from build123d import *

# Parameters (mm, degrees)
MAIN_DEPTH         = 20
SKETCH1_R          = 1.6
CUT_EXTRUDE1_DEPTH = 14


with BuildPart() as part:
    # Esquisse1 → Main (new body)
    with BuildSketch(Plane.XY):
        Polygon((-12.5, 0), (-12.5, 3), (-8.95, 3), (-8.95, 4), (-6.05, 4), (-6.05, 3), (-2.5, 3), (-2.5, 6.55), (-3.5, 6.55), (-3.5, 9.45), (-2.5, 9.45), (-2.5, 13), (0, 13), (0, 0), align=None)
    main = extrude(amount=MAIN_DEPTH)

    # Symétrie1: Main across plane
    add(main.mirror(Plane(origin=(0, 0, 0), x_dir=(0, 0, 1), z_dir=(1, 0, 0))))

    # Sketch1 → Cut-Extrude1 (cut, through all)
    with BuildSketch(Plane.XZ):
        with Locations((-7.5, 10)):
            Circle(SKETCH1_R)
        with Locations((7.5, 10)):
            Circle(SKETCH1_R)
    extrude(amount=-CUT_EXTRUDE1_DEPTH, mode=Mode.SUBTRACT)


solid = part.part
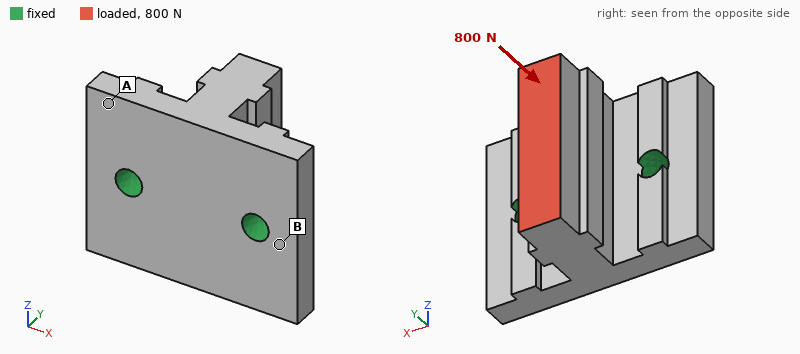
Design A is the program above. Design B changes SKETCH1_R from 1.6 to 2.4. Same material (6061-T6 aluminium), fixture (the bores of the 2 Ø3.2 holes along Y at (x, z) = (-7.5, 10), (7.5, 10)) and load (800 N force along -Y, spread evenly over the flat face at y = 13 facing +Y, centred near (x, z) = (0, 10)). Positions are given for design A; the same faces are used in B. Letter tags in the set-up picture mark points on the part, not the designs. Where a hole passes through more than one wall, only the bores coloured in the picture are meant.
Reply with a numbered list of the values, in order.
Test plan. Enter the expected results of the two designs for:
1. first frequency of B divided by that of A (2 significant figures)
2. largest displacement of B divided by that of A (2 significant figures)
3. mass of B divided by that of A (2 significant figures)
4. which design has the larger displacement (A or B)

1. 1.2
2. 0.75
3. 0.97
4. A
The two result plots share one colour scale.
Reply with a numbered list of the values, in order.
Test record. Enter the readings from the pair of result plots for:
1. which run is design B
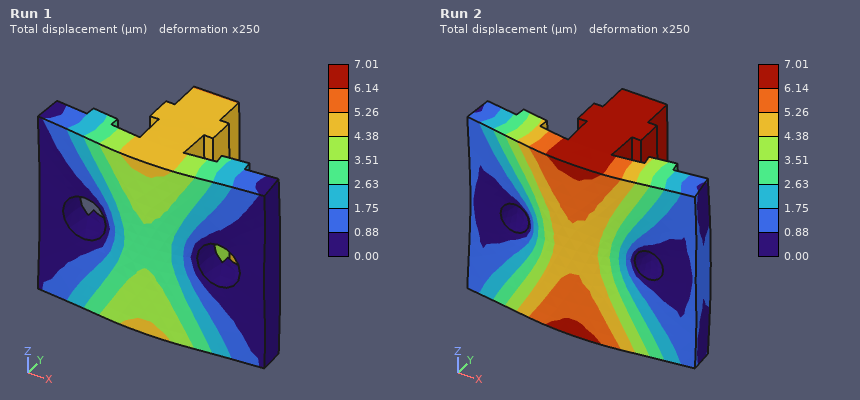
1. Run 1
